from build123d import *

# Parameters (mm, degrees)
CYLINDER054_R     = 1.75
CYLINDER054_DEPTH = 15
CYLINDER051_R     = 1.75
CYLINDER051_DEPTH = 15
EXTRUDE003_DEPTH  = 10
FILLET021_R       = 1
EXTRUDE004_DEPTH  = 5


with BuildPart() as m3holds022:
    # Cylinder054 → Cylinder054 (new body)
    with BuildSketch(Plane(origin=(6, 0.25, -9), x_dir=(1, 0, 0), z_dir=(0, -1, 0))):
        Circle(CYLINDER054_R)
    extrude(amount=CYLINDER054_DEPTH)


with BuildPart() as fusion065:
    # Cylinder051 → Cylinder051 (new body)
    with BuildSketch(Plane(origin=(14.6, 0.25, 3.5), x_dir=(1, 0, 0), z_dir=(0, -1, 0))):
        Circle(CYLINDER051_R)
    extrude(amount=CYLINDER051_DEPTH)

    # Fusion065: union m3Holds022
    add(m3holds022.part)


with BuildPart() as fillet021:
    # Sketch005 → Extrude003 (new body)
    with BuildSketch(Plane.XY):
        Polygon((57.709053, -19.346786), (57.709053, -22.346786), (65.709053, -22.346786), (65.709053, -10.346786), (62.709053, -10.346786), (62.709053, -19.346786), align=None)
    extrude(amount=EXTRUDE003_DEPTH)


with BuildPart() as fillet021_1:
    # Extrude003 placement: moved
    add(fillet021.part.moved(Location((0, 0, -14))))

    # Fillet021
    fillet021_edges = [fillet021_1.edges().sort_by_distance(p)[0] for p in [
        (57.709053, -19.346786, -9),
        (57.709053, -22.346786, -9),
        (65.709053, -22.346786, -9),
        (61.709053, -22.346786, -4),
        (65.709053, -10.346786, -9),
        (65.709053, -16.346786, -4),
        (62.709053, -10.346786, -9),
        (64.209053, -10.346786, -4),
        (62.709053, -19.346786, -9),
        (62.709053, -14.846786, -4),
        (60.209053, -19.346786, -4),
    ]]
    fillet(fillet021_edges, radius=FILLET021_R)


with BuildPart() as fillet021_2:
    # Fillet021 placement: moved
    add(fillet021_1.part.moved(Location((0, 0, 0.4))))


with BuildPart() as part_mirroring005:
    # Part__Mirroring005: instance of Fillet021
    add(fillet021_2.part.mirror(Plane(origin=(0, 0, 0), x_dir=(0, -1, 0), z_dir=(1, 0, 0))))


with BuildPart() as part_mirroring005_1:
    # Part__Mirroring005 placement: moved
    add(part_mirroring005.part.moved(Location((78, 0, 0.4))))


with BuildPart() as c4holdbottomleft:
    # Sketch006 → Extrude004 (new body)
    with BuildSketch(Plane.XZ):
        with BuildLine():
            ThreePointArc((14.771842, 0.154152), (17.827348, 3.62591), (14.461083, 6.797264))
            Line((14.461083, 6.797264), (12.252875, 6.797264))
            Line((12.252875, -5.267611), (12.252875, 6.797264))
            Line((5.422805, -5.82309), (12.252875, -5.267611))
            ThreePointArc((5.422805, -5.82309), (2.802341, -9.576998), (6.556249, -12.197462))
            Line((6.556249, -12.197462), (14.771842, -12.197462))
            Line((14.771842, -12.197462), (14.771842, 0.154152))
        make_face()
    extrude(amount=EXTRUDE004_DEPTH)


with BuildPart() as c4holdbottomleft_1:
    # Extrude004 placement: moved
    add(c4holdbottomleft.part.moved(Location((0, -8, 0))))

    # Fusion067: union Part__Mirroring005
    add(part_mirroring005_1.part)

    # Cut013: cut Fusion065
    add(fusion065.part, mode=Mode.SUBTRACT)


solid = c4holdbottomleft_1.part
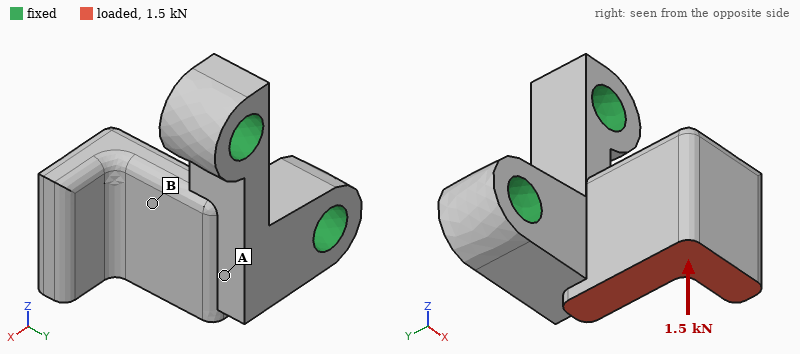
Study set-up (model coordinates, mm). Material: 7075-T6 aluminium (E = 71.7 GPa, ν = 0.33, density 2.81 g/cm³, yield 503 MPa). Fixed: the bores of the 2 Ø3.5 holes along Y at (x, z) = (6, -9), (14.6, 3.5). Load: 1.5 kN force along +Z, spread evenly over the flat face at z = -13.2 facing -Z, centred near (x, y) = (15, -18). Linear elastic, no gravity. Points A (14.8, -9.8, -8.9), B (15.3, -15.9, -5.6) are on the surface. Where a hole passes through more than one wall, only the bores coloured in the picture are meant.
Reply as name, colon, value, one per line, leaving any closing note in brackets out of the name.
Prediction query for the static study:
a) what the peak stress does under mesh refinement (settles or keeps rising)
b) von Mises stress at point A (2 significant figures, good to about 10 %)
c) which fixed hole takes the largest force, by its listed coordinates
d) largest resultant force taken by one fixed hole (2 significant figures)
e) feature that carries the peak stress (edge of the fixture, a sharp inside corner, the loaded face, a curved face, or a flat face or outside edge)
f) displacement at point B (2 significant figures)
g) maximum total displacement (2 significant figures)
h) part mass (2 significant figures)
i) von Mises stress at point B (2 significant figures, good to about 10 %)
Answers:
what the peak stress does under mesh refinement: keeps rising
von Mises stress at point A: 51 MPa
which fixed hole takes the largest force, by its listed coordinates: (14.6, 3.5)
largest resultant force taken by one fixed hole: 1.4 kN
feature that carries the peak stress: a sharp inside corner
displacement at point B: 0.055 mm
maximum total displacement: 0.15 mm
part mass: 2.7 g
von Mises stress at point B: 170 MPa
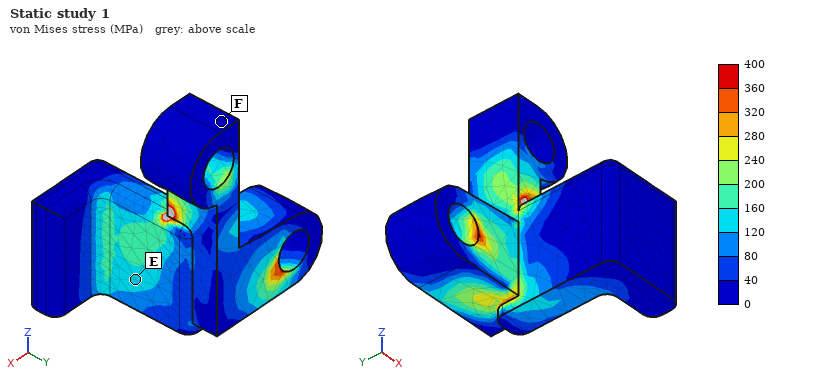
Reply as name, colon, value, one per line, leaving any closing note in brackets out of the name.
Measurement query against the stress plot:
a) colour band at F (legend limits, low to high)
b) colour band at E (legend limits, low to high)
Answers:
colour band at F: 0 to 40 MPa
colour band at E: 120 to 160 MPa
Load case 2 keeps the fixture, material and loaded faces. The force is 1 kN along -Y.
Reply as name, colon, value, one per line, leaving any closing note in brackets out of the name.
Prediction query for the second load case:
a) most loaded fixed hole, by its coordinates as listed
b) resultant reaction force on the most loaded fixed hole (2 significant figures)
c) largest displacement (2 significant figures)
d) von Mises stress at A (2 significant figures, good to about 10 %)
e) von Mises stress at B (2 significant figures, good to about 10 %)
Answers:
most loaded fixed hole, by its coordinates as listed: (6, -9)
resultant reaction force on the most loaded fixed hole: 1.0 kN
largest displacement: 0.20 mm
von Mises stress at A: 83 MPa
von Mises stress at B: 66 MPa
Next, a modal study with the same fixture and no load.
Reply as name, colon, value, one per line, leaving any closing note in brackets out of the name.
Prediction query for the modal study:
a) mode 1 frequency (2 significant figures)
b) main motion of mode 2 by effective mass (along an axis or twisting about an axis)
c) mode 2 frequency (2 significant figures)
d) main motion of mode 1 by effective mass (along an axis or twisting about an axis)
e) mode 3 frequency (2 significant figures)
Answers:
mode 1 frequency: 9500 Hz
main motion of mode 2 by effective mass: along Z
mode 2 frequency: 17 kHz
main motion of mode 1 by effective mass: along X
mode 3 frequency: 26 kHz
